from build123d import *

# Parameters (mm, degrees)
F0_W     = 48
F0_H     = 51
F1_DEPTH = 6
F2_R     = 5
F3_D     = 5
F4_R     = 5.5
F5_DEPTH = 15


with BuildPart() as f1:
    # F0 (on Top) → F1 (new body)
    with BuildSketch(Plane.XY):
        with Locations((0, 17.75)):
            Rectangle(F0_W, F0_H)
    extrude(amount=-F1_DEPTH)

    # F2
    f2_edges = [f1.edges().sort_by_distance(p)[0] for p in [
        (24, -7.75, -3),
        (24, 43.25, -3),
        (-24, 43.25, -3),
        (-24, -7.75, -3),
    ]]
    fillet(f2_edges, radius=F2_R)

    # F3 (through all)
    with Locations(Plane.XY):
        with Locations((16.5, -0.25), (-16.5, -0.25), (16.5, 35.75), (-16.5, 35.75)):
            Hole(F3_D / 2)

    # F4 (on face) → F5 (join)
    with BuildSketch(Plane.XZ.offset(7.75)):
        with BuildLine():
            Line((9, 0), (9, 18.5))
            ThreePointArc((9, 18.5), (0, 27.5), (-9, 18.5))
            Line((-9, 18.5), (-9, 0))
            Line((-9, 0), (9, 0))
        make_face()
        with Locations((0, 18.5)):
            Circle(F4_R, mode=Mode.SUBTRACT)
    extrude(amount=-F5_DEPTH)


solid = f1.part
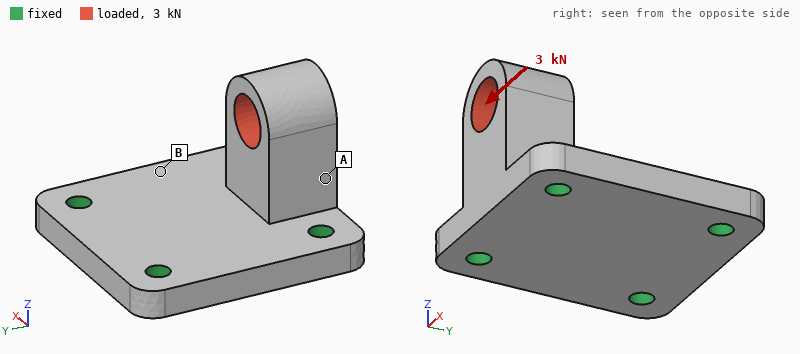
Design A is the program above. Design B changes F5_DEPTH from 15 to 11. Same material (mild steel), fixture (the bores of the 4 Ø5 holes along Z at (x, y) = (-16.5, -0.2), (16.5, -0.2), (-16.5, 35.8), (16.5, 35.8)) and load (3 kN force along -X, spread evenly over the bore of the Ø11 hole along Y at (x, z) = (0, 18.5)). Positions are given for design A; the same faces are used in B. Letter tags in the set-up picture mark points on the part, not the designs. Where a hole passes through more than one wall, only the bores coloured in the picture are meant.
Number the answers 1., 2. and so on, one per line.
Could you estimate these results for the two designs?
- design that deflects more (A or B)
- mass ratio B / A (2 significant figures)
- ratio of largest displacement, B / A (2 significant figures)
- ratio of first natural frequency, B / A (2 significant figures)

1. B
2. 0.93
3. 1.3
4. 0.94
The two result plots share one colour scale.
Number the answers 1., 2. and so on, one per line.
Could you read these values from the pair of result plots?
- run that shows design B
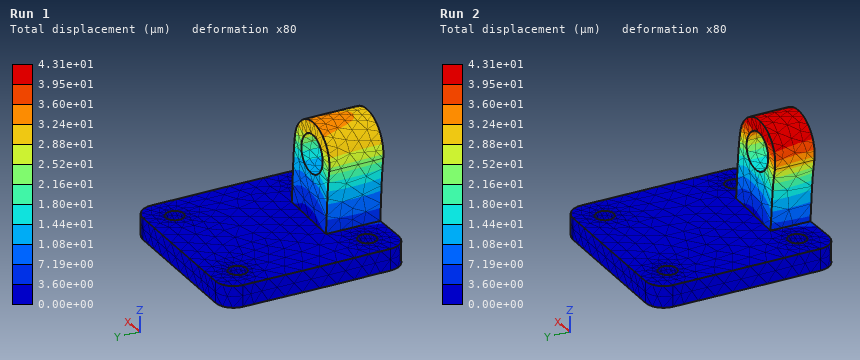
1. Run 2
